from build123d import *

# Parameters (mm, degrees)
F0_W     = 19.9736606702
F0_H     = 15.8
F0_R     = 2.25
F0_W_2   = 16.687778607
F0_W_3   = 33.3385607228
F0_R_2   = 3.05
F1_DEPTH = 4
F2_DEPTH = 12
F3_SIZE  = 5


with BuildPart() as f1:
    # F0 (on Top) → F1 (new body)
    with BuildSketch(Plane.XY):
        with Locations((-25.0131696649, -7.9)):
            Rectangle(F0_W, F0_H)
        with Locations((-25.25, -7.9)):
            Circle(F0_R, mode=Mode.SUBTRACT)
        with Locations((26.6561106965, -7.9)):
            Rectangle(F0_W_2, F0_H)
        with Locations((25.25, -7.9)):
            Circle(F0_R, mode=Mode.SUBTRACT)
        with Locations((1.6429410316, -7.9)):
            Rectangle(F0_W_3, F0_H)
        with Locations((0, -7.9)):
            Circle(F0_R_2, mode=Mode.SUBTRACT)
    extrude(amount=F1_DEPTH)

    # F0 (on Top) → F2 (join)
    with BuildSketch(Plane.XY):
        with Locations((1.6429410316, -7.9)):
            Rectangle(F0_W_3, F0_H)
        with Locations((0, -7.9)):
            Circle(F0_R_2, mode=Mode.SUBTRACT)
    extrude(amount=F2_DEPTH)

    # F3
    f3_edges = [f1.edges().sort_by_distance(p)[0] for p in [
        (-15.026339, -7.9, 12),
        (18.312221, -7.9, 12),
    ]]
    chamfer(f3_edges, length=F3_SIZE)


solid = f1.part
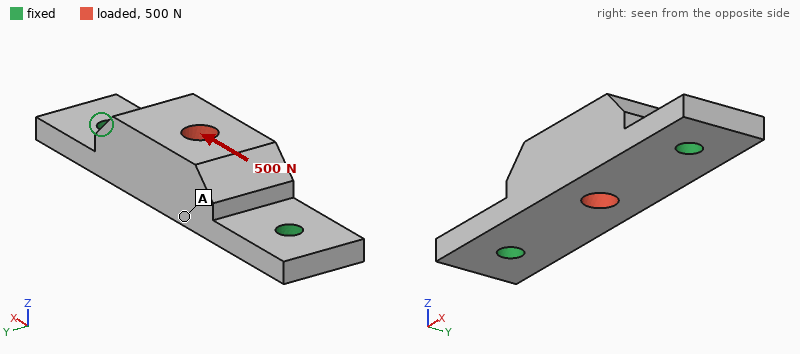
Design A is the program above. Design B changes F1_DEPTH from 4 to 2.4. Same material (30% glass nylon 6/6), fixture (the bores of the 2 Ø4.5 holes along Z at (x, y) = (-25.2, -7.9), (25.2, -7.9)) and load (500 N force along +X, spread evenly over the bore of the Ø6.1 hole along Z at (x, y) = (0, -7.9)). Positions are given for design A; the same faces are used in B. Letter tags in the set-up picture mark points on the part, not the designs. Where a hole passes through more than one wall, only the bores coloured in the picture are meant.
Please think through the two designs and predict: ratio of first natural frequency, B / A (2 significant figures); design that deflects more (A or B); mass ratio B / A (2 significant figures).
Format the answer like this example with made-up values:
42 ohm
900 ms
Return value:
0.55
B
0.89
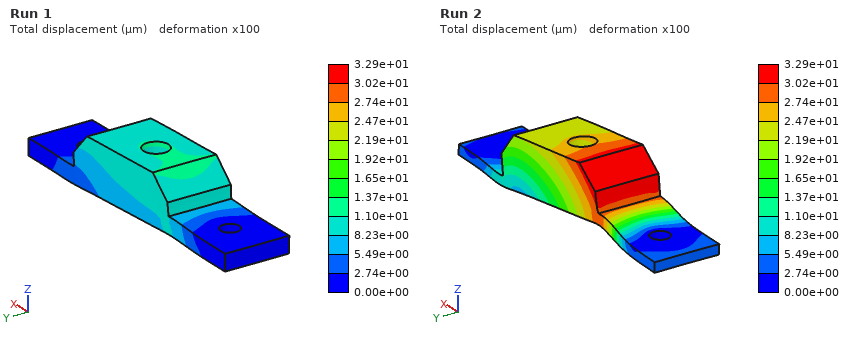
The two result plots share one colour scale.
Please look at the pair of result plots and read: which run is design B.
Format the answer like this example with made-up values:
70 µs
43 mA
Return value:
Run 2
